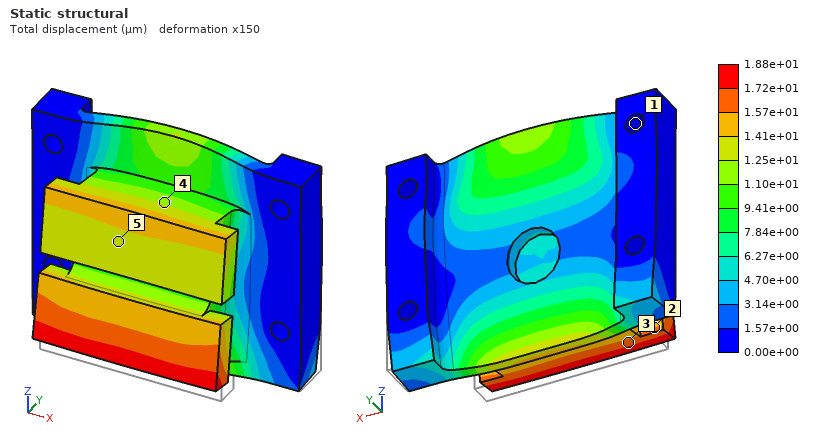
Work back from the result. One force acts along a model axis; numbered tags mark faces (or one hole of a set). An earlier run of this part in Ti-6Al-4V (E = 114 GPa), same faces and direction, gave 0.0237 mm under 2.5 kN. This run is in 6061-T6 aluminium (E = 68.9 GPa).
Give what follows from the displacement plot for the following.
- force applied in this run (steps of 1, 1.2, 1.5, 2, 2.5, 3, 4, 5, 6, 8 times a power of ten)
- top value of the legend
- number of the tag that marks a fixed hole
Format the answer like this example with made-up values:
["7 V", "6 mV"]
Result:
["1.2 kN", "1.88e+01 µm", "1"]
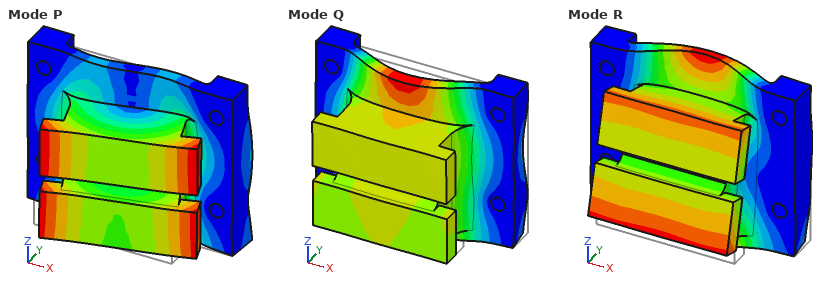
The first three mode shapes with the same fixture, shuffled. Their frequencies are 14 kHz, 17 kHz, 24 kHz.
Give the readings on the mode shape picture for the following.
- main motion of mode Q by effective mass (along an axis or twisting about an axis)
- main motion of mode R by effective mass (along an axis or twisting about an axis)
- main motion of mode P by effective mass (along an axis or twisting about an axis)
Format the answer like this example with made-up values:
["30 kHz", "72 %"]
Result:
["along Y", "along Z", "along X"]
